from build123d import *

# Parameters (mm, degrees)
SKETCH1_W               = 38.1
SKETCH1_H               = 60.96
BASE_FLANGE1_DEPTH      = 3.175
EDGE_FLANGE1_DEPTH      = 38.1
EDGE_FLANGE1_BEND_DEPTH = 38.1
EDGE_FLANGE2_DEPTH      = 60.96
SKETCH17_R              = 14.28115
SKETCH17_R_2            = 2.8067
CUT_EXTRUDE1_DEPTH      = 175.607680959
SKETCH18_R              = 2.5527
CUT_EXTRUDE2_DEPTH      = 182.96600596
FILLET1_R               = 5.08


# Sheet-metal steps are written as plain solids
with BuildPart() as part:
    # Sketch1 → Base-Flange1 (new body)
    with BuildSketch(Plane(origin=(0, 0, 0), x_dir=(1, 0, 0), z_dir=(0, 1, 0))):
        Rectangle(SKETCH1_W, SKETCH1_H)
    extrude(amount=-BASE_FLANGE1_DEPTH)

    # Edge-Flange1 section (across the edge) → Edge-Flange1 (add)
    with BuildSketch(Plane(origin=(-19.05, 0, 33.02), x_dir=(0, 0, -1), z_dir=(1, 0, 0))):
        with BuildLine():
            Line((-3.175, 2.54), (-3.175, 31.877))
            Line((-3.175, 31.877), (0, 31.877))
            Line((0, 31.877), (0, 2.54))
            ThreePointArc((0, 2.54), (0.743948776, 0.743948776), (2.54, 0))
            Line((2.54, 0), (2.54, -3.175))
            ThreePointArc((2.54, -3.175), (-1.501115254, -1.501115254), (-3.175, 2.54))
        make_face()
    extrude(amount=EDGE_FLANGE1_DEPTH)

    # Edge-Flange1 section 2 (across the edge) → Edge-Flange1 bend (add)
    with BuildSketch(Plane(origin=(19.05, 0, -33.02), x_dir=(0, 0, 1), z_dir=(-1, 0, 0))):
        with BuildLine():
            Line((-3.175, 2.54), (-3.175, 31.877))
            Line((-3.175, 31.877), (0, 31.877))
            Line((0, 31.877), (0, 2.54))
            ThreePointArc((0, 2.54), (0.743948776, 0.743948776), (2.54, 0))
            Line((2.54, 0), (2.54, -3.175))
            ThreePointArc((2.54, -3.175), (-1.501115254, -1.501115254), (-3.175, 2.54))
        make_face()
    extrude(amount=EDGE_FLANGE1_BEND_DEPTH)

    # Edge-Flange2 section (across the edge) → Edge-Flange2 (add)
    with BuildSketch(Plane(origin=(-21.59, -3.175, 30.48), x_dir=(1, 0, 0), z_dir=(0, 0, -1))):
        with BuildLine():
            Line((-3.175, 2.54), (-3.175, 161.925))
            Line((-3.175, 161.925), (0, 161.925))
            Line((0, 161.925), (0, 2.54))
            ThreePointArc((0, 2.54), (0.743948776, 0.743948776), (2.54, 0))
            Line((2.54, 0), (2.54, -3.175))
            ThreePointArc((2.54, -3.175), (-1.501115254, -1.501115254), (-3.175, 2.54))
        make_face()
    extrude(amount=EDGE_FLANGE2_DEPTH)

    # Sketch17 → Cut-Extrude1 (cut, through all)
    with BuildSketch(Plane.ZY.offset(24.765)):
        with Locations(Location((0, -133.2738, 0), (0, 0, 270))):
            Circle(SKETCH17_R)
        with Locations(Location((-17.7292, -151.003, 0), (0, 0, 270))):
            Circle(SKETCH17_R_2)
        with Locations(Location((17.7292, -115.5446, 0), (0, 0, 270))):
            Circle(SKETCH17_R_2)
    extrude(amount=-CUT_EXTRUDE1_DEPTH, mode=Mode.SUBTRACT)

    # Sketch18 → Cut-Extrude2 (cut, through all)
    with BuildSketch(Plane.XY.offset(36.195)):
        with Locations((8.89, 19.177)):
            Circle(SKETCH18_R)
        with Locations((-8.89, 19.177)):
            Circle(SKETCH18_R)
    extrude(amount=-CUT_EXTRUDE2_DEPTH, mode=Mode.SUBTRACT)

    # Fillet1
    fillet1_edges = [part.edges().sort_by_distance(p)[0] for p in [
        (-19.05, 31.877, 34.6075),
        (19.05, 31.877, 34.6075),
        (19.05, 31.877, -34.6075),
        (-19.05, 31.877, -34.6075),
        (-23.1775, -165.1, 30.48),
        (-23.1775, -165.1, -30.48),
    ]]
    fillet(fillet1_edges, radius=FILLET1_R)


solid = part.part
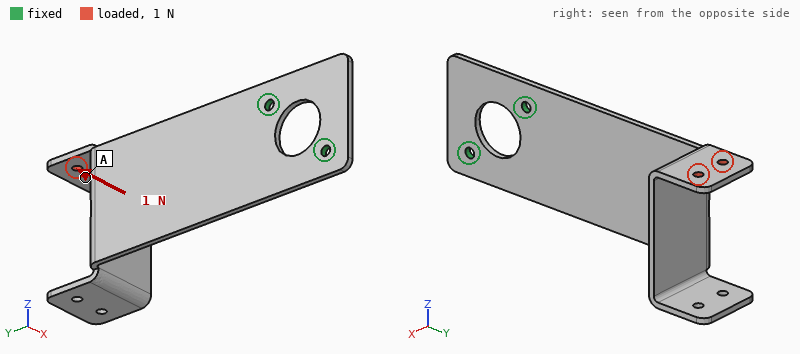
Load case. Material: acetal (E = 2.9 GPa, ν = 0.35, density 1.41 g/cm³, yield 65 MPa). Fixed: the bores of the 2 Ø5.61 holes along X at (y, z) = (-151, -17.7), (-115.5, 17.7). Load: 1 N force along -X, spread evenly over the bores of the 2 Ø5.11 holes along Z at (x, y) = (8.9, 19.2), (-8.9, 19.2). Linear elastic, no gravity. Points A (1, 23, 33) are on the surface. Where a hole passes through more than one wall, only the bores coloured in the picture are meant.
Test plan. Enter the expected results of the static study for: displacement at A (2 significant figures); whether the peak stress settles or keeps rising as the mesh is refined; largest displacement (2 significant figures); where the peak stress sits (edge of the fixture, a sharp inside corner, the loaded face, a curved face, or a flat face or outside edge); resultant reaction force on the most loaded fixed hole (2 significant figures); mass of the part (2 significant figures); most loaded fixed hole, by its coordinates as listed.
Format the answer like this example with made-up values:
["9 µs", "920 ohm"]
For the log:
["2.1 mm", "keeps rising", "2.4 mm", "edge of the fixture", "2.3 N", "64 g", "(-115.5, 17.7)"]
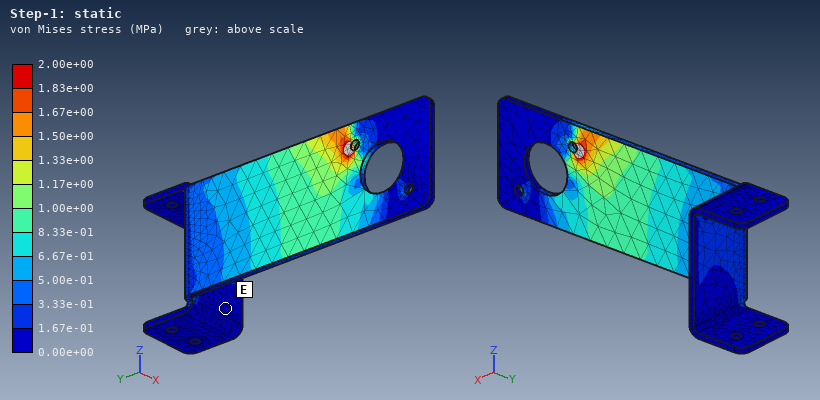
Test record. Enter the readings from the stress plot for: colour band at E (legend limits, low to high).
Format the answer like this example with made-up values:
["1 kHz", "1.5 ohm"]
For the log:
["0.00e+00 to 1.67e-01 MPa"]
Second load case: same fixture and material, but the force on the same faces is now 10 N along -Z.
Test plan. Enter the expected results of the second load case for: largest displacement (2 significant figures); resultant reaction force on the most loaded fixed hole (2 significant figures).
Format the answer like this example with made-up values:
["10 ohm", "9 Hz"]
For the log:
["2.5 mm", "33 N"]
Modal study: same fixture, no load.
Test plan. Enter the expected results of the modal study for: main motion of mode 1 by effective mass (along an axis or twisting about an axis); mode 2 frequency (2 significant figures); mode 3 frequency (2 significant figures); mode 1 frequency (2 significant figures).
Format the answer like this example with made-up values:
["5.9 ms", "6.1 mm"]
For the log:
["along X", "65 Hz", "130 Hz", "24 Hz"]
